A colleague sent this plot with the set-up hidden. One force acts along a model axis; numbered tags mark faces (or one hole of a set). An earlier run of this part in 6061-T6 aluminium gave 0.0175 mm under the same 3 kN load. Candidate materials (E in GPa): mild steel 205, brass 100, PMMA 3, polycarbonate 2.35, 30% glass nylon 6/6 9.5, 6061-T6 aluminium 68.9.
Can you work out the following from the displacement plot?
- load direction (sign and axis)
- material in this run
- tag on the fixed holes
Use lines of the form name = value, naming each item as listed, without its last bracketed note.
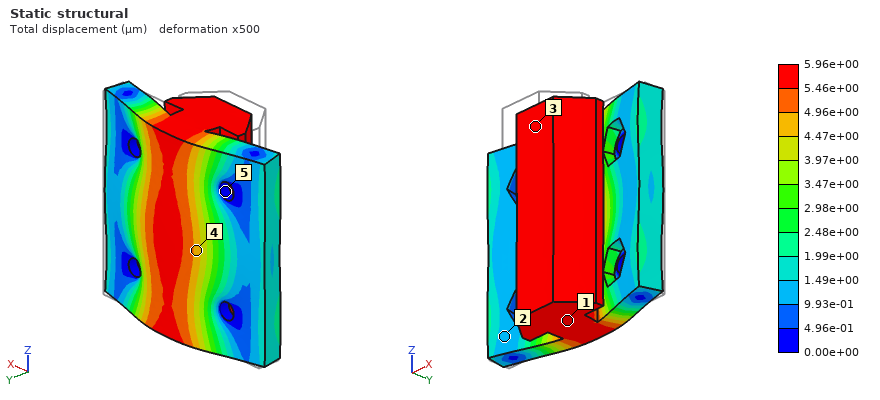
load direction = +Y
material in this run = mild steel
tag on the fixed holes = 5
